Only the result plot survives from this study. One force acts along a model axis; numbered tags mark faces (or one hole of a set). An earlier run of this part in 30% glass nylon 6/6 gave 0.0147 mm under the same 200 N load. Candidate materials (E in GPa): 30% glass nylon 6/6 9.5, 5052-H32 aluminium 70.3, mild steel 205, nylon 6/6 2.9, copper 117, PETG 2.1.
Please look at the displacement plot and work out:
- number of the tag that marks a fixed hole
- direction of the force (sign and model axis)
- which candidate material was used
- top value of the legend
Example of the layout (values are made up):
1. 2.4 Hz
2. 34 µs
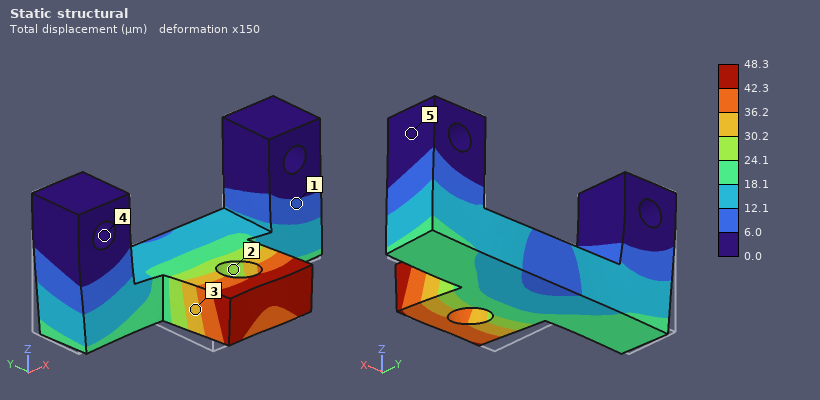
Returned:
1. 4
2. +X
3. nylon 6/6
4. 48.3 µm
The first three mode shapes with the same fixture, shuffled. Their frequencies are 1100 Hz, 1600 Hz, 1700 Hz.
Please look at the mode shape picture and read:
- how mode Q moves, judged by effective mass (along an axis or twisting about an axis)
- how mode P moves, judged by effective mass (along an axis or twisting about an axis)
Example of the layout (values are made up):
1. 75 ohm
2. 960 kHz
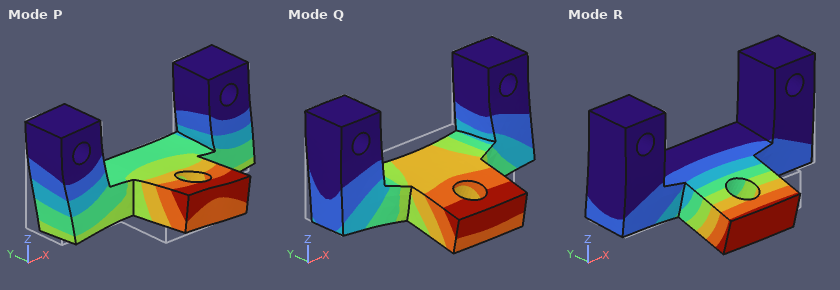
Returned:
1. along Y
2. along X
